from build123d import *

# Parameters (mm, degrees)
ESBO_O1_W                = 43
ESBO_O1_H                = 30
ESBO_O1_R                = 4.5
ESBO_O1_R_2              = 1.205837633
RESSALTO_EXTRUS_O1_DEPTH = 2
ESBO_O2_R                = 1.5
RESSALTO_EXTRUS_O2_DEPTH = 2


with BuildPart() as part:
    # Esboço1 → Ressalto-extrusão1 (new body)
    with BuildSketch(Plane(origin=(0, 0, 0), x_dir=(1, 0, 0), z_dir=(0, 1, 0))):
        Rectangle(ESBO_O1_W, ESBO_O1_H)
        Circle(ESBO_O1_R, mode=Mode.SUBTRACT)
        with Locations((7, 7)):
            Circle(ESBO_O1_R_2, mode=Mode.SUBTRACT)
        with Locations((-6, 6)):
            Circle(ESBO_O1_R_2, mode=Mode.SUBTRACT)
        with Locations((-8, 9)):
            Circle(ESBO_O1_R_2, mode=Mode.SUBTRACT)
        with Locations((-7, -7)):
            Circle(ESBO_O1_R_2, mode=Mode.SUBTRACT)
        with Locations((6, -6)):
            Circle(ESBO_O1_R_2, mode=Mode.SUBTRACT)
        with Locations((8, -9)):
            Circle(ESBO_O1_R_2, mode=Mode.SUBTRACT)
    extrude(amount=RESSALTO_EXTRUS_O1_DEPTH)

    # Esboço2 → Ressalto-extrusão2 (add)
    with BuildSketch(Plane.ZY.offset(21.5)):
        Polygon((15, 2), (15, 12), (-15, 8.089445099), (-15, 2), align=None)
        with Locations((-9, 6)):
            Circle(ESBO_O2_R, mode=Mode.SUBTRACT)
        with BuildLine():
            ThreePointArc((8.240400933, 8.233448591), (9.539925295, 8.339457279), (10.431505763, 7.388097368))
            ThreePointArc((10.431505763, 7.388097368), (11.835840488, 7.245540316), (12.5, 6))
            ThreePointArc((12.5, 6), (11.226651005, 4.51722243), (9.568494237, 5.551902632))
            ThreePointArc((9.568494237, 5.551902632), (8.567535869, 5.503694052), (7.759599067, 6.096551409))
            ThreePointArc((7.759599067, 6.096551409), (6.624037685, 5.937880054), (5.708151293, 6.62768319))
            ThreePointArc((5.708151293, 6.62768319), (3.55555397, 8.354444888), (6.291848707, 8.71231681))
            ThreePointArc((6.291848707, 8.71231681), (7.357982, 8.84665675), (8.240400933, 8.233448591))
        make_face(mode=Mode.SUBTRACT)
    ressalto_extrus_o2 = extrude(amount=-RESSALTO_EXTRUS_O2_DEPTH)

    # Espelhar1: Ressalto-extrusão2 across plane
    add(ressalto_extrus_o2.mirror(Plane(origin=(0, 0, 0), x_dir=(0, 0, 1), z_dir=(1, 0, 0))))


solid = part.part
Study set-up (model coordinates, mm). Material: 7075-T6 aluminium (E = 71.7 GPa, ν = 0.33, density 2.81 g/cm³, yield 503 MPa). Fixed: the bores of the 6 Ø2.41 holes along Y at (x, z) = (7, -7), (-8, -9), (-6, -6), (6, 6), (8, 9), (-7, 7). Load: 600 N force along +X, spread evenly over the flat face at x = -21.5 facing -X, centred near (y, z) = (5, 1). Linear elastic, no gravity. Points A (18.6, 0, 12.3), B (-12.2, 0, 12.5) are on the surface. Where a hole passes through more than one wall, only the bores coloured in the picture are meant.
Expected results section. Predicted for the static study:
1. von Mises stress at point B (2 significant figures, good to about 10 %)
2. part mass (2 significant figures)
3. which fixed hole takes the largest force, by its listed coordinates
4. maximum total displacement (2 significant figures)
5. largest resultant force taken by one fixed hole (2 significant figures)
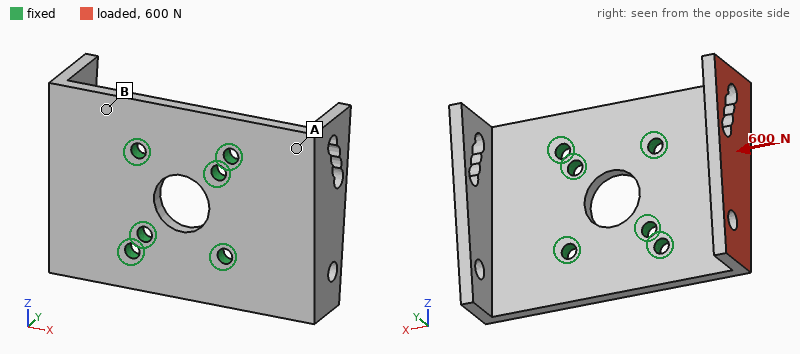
100 MPa
9.1 g
(-7, 7)
0.36 mm
270 N
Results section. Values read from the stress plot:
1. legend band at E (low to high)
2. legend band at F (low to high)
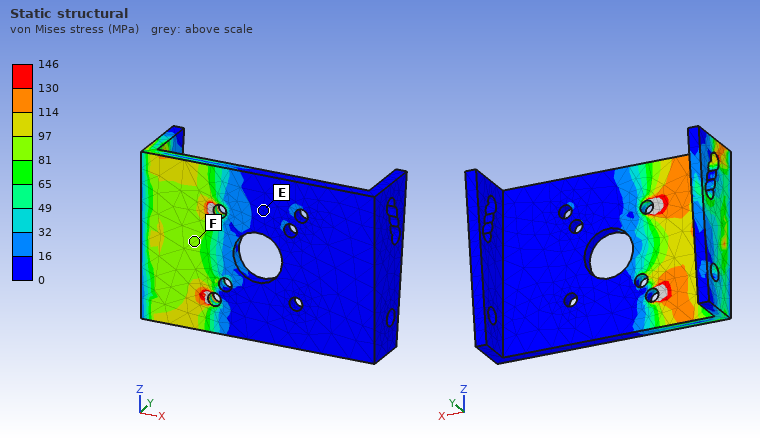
0 to 16 MPa
81 to 97 MPa
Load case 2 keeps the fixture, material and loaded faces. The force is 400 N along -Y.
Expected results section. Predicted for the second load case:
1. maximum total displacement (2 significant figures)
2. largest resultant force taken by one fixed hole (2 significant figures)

0.43 mm
280 N
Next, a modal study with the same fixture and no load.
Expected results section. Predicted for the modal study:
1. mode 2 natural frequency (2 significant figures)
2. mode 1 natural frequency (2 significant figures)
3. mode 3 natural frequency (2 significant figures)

4500 Hz
4500 Hz
7100 Hz
